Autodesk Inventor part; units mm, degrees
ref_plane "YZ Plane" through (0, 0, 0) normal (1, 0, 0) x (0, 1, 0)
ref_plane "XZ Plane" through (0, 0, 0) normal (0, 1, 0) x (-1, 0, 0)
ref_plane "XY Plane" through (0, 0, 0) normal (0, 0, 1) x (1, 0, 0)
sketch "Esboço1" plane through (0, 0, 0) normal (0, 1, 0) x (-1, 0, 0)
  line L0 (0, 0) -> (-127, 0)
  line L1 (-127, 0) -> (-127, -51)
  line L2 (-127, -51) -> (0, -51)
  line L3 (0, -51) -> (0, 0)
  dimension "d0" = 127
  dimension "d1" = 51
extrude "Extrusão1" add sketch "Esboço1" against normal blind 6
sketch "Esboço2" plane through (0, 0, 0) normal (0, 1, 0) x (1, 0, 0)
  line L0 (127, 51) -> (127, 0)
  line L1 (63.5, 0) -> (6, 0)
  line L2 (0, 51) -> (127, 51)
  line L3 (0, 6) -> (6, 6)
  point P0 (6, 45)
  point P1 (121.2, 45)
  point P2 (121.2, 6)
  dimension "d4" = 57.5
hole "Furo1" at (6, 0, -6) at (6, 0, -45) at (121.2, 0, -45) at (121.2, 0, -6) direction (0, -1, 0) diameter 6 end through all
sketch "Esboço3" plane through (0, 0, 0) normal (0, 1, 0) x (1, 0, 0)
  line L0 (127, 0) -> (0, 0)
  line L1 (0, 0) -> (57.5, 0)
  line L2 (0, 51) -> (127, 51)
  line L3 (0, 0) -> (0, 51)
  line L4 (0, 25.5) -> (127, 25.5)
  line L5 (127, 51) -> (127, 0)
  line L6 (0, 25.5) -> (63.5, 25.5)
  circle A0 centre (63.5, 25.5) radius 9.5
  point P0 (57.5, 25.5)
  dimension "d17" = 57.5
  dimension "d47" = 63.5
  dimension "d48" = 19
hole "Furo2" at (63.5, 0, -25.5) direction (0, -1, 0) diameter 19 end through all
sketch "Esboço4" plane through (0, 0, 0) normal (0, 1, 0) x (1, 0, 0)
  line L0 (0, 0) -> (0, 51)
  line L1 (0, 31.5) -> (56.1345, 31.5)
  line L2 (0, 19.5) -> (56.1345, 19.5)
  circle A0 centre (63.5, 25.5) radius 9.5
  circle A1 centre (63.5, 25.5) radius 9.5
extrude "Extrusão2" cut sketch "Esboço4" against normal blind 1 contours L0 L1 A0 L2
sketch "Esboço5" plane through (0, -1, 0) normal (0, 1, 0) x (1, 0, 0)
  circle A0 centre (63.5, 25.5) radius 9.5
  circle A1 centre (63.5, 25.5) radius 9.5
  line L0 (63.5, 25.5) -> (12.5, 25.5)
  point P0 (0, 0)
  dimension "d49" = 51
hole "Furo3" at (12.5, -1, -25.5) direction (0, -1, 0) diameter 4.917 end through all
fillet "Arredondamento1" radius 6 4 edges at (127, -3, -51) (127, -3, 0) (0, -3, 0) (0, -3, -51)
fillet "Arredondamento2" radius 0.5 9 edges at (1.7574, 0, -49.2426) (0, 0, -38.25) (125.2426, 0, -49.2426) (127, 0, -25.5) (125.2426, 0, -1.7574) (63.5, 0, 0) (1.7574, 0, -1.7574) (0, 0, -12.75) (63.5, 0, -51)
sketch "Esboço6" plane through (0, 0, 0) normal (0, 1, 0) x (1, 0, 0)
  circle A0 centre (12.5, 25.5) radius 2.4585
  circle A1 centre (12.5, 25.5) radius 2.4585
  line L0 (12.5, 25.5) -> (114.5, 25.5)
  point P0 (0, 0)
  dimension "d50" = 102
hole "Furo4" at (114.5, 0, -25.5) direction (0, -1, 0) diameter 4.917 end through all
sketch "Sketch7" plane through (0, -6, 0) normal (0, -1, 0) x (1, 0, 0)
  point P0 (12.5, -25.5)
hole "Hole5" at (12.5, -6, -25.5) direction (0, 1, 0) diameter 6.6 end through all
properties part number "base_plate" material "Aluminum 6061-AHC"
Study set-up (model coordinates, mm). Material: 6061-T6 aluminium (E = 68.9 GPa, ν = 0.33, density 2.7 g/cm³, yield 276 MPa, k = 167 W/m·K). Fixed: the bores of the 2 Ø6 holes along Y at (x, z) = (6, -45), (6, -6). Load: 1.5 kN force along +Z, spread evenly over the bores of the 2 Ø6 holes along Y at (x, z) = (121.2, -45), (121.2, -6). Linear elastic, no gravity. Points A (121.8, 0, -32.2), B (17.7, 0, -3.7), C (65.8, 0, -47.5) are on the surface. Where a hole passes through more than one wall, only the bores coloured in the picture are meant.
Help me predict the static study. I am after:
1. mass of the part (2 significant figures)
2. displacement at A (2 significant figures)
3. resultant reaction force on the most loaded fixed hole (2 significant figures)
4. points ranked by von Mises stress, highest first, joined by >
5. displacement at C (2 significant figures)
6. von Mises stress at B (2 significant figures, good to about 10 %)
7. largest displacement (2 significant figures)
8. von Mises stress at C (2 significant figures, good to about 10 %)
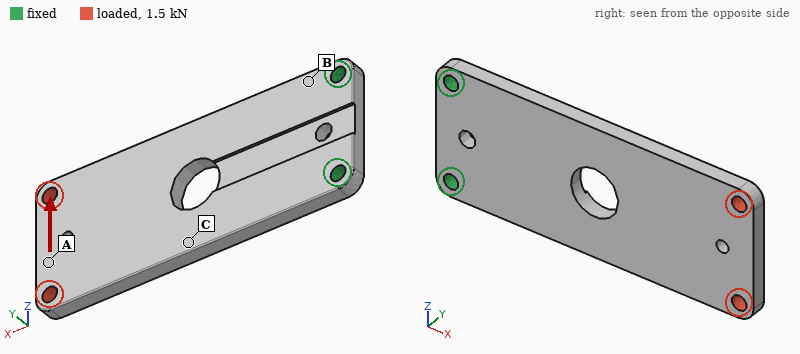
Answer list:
95 g
0.21 mm
4.3 kN
B > C > A
0.087 mm
53 MPa
0.22 mm
28 MPa
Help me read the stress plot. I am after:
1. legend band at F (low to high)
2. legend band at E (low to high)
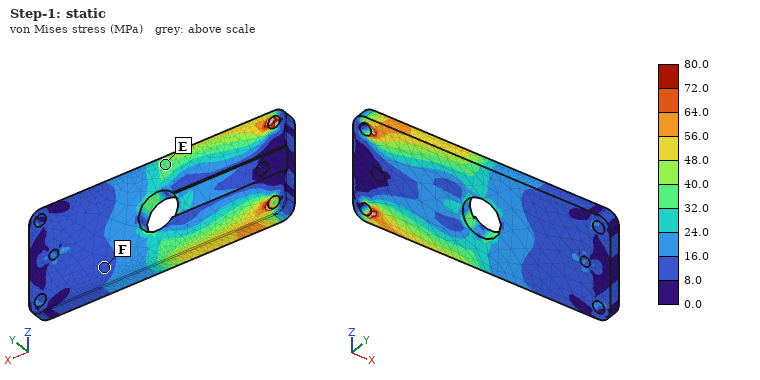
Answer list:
8.0 to 16.0 MPa
32.0 to 40.0 MPa
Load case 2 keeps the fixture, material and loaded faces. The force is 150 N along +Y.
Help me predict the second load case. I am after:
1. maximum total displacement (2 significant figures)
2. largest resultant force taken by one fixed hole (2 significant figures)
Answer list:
1.5 mm
98 N
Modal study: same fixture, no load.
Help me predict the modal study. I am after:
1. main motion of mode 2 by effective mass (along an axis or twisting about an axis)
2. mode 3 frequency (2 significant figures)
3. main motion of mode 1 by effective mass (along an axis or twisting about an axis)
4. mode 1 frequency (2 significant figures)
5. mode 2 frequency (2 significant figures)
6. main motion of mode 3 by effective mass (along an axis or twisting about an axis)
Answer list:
twisting about X
2000 Hz
along Y
320 Hz
1500 Hz
along Y
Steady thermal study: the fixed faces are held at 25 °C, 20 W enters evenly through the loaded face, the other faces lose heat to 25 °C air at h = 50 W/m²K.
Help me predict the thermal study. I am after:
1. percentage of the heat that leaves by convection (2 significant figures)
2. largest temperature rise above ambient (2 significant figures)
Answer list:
53 %
36 K
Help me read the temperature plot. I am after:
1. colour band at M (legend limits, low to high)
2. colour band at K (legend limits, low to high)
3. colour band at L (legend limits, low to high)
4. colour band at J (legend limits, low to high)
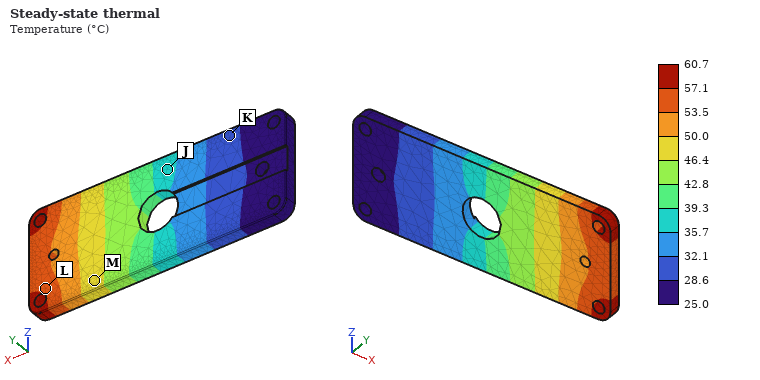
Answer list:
46.4 to 50.0 °C
28.6 to 32.1 °C
53.5 to 57.1 °C
35.7 to 39.3 °C
